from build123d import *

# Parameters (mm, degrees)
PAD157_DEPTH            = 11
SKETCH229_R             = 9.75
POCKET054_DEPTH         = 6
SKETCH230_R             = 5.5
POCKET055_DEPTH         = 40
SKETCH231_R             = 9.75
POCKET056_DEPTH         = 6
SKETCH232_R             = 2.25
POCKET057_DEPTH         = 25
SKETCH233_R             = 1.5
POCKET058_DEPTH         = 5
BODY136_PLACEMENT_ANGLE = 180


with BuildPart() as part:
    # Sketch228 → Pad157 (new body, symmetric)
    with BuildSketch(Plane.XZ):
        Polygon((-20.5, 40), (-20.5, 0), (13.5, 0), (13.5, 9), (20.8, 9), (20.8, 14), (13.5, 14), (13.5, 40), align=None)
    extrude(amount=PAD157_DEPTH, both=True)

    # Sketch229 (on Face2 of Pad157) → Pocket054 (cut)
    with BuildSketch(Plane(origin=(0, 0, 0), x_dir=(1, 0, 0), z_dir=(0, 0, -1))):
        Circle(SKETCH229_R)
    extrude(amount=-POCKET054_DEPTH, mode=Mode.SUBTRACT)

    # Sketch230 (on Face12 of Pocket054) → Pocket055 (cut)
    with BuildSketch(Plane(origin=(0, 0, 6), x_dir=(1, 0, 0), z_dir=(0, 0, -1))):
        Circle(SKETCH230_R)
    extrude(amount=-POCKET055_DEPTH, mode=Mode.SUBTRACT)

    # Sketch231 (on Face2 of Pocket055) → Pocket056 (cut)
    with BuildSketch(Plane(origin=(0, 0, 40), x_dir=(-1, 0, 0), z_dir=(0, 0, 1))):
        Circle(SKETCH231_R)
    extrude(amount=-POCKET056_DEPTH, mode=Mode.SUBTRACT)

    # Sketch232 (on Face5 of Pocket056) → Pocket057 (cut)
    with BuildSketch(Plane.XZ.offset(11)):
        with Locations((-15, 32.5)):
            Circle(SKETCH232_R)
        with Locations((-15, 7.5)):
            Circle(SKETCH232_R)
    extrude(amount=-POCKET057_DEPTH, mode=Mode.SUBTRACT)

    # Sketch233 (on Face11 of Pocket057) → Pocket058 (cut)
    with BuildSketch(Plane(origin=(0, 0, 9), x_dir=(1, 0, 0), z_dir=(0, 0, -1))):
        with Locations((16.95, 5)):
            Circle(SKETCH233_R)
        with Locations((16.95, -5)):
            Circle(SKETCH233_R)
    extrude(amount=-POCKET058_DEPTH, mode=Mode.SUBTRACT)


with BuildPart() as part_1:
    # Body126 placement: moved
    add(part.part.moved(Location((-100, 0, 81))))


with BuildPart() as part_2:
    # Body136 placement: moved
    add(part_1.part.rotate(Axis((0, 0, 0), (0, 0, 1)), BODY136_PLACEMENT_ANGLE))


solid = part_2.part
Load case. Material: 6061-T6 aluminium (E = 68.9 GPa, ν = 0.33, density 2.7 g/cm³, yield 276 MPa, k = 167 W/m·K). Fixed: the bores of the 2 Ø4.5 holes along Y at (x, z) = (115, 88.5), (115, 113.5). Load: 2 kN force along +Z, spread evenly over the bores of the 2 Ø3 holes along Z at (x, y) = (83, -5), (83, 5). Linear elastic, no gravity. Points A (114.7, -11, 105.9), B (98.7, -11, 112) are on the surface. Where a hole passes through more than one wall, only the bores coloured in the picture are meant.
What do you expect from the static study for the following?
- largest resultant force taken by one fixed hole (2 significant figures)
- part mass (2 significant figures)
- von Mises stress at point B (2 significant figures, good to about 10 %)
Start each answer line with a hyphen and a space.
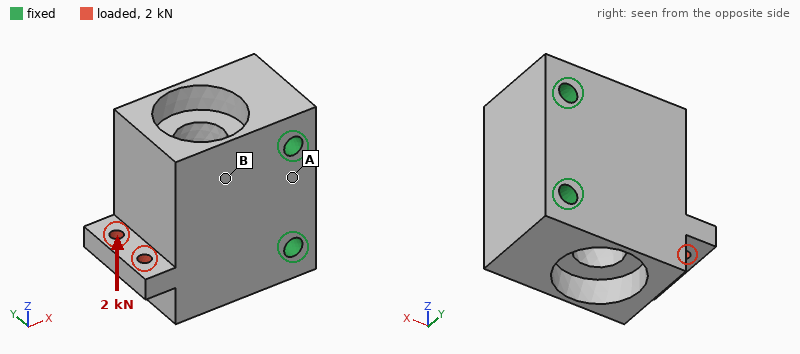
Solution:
- 2.6 kN
- 64 g
- 12 MPa
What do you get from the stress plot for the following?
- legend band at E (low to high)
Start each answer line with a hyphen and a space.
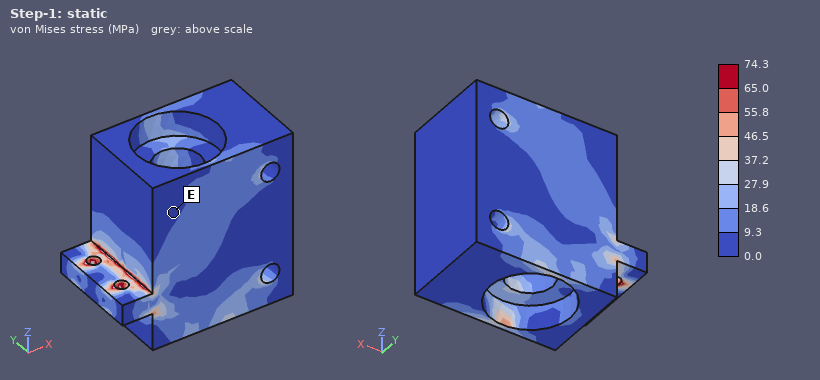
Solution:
- 0.0 to 9.3 MPa
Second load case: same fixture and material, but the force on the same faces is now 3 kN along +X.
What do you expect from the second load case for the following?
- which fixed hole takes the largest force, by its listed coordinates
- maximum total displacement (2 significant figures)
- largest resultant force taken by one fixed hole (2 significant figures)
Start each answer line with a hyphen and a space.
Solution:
- (115, 88.5)
- 12 µm
- 2.5 kN
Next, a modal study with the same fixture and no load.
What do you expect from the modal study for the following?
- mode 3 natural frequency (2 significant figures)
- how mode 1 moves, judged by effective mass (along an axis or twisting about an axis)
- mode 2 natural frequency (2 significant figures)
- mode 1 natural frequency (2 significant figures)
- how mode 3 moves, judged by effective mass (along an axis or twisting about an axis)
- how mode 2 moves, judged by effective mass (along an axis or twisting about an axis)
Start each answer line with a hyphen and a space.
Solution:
- 17 kHz
- along Y
- 16 kHz
- 11 kHz
- twisting about X
- along Z
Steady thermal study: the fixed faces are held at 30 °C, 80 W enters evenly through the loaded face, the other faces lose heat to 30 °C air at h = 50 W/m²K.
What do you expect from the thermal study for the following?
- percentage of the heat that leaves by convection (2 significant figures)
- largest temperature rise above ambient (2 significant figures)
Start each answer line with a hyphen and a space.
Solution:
- 6.8 %
- 64 K
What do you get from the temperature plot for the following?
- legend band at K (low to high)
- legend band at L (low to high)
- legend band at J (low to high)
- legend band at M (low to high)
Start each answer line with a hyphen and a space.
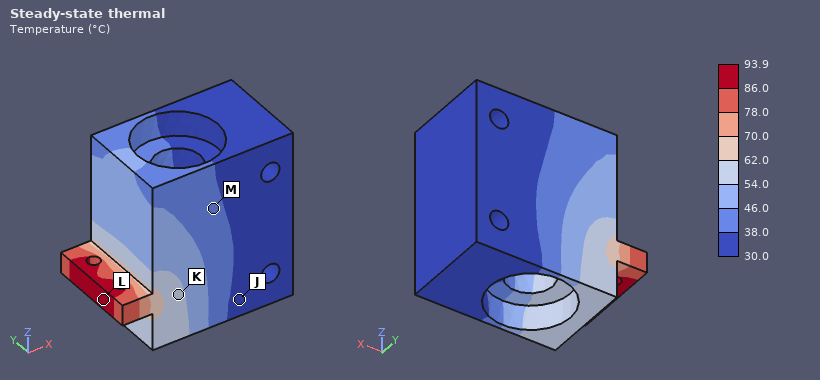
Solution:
- 54.0 to 62.0 °C
- 86.0 to 93.9 °C
- 30.0 to 38.0 °C
- 38.0 to 46.0 °C
